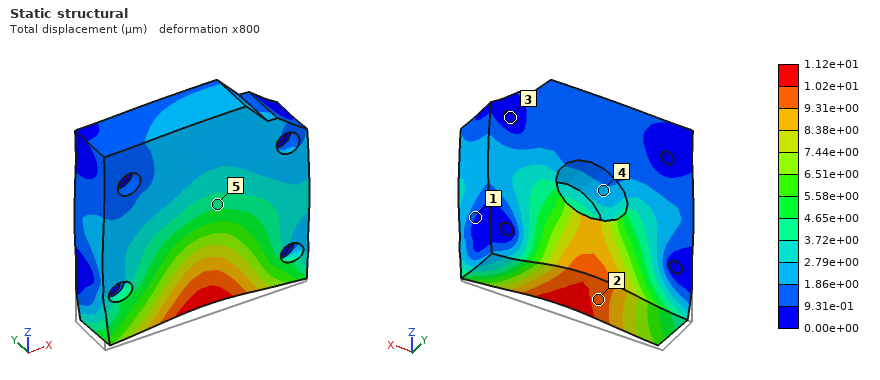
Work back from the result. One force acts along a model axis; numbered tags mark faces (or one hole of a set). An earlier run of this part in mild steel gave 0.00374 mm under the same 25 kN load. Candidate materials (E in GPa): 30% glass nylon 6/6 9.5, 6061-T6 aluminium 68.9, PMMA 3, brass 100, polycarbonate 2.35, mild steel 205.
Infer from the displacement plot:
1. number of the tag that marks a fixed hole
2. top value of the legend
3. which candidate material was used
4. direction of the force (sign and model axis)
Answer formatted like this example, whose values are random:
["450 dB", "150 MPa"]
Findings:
["3", "1.12e+01 µm", "6061-T6 aluminium", "+Z"]
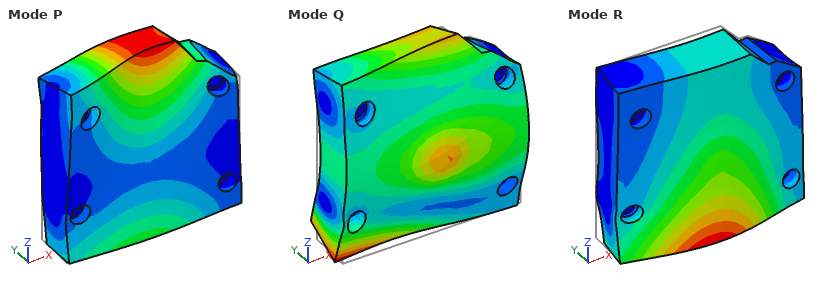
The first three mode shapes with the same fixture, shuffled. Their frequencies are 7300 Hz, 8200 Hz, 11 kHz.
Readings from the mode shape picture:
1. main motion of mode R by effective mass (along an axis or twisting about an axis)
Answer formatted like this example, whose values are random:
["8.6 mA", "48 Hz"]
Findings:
["along Y"]
